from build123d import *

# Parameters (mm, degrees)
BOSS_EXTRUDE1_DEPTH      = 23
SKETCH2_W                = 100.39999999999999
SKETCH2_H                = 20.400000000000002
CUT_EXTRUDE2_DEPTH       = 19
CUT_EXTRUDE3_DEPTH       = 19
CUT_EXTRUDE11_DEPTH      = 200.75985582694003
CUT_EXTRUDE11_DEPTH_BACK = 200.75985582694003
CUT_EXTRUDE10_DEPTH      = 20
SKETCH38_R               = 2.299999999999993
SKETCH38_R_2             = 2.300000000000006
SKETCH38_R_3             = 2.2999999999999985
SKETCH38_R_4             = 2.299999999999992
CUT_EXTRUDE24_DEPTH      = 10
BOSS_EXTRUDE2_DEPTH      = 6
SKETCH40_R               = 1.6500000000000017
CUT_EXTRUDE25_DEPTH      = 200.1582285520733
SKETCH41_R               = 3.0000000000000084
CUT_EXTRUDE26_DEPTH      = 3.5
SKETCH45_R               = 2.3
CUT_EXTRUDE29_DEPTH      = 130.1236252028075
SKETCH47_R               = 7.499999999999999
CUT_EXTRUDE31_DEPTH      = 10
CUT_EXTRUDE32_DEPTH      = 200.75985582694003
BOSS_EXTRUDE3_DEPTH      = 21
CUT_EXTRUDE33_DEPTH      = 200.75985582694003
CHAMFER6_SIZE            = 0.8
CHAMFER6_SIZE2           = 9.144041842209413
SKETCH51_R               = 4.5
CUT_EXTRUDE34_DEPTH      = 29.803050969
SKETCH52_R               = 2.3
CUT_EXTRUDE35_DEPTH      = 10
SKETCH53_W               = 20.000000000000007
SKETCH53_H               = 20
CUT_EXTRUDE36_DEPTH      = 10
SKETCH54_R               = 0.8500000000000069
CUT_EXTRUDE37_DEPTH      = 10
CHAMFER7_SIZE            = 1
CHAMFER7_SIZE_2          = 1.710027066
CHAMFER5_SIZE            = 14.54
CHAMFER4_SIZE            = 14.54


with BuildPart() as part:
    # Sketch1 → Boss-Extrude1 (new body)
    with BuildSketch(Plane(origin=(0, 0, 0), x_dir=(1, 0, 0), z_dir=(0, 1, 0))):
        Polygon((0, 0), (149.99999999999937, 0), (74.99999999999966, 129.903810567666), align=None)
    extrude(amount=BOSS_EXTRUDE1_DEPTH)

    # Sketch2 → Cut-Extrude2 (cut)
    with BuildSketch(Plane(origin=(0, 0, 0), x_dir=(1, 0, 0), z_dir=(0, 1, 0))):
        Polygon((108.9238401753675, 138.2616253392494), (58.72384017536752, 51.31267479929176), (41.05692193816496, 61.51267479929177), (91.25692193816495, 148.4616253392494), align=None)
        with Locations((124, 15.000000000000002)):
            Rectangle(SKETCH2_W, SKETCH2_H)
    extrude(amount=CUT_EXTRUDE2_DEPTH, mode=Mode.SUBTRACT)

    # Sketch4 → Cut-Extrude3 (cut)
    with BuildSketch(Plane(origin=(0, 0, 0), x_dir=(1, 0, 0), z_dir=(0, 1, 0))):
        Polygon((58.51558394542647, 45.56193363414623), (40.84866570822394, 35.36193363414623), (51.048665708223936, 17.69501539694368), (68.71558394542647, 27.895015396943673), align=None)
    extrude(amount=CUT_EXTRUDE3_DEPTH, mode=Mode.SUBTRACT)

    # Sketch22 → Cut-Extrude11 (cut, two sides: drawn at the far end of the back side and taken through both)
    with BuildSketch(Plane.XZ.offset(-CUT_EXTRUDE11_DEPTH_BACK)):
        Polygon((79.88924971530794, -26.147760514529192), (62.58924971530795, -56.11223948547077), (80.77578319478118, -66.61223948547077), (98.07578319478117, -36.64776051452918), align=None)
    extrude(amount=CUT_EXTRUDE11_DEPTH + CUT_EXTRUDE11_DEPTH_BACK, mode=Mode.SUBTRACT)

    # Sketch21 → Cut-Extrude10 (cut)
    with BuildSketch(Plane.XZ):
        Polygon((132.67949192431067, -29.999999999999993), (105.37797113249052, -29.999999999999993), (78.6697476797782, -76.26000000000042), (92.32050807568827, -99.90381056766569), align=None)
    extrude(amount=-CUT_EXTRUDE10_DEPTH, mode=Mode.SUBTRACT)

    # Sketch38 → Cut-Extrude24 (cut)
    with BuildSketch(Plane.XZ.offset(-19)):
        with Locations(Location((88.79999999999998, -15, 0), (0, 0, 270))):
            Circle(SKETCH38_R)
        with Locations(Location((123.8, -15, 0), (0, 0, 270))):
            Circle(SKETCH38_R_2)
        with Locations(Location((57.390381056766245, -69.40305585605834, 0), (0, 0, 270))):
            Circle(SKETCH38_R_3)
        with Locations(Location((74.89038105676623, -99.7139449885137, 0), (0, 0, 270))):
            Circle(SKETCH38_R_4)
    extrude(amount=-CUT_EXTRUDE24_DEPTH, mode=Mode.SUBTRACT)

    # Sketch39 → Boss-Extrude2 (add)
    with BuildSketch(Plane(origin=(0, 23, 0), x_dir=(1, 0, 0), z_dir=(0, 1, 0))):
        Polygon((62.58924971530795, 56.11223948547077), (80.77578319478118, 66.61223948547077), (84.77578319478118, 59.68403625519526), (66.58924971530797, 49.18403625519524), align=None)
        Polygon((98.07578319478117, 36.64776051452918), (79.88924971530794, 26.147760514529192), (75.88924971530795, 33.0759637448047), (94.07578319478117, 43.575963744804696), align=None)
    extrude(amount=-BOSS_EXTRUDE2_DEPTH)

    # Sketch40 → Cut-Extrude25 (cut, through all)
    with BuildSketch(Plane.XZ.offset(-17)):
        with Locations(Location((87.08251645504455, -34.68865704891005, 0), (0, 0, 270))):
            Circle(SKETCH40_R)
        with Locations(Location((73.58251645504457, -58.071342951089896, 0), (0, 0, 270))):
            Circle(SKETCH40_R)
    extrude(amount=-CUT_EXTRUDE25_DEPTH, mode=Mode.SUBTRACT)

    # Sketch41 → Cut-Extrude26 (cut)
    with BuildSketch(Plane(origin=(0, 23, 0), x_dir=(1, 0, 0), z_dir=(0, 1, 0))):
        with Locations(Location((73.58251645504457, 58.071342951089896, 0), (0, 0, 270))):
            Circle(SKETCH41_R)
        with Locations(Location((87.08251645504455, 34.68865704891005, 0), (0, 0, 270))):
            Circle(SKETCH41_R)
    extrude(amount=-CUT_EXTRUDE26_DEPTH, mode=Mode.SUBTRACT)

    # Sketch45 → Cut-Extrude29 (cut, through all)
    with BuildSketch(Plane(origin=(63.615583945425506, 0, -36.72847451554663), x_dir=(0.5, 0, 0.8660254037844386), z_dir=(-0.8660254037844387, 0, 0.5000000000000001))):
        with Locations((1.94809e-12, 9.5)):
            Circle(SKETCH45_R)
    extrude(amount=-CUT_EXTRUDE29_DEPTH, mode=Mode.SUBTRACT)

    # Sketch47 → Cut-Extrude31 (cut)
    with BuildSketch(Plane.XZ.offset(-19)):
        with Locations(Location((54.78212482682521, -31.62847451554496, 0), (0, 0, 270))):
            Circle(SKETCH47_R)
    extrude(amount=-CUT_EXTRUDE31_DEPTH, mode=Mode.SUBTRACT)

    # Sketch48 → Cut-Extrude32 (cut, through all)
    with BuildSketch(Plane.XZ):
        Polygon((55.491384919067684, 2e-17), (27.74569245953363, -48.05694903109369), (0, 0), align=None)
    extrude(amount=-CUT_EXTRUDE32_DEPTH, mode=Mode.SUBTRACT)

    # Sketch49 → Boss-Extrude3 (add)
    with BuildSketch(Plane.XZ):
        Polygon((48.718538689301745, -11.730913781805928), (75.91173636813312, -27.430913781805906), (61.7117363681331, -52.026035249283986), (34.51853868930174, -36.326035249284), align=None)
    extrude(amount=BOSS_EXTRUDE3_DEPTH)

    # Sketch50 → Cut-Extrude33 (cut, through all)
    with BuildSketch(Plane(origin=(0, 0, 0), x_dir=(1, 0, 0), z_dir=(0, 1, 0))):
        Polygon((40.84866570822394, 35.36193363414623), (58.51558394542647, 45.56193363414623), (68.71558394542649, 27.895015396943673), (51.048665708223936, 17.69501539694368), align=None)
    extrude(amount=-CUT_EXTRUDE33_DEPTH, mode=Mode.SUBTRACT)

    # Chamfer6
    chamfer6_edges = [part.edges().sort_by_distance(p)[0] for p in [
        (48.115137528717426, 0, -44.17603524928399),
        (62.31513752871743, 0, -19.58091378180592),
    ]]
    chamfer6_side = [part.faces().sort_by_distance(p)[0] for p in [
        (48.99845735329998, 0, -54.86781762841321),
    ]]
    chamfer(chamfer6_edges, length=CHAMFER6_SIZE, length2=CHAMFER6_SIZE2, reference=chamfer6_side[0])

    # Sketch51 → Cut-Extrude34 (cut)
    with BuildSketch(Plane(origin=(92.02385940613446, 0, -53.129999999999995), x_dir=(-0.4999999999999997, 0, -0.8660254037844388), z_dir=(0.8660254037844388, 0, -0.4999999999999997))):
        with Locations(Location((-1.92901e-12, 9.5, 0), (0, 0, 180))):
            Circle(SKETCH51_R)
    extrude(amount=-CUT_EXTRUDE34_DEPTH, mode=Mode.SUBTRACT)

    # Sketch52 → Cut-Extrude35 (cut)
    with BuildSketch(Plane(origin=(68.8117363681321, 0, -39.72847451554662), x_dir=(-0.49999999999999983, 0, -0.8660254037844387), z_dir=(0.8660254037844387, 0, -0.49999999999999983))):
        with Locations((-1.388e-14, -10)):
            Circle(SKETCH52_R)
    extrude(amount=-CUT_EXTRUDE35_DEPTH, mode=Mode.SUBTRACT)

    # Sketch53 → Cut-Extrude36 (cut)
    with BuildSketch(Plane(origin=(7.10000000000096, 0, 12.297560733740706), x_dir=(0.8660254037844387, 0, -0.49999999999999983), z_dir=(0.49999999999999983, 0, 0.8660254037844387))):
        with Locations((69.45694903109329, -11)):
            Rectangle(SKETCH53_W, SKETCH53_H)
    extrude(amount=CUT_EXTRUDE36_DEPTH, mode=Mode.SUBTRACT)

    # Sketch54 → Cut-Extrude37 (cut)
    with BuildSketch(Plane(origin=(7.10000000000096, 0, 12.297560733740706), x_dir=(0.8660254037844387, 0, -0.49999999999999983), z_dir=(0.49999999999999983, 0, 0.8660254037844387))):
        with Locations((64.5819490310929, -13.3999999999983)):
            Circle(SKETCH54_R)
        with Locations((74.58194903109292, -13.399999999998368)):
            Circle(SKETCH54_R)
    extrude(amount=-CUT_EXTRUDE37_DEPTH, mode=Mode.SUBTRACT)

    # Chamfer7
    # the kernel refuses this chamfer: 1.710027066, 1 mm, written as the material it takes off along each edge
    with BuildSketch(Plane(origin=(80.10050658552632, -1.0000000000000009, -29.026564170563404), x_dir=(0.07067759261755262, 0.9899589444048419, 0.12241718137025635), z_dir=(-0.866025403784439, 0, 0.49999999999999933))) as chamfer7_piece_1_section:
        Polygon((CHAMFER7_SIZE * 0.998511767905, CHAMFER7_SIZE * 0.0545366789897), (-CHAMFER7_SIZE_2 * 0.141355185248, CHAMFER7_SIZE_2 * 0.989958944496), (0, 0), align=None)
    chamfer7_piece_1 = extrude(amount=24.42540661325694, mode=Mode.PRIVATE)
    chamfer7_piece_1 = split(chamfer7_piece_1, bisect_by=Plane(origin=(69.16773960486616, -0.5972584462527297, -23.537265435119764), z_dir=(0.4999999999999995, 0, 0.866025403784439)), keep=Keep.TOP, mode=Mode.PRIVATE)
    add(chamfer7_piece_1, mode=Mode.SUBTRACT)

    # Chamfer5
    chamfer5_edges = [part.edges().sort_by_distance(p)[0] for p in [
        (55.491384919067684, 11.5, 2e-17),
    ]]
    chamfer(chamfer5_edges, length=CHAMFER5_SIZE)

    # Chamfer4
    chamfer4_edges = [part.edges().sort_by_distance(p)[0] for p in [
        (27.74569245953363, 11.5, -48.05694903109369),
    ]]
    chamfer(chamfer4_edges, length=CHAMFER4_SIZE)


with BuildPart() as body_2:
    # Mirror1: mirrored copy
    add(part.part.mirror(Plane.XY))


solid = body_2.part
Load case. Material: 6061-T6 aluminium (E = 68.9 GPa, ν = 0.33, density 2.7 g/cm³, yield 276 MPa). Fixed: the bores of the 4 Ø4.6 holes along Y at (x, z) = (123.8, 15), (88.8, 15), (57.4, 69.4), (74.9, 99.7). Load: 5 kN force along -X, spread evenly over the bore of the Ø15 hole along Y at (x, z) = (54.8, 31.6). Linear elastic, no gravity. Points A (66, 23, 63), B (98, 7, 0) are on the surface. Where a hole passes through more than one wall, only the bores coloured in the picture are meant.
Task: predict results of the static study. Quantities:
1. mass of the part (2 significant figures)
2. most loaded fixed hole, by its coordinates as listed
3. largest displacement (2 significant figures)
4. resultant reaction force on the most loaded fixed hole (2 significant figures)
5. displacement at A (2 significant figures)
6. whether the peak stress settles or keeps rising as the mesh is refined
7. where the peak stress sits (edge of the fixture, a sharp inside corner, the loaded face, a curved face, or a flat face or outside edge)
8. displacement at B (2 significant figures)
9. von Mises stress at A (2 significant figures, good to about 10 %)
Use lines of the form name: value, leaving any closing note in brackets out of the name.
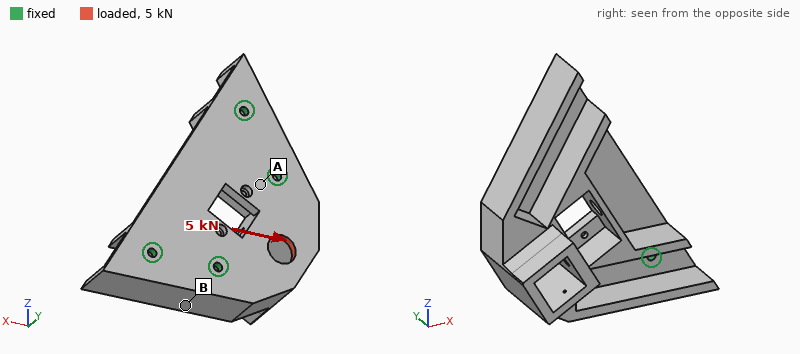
mass of the part: 240 g
most loaded fixed hole, by its coordinates as listed: (88.8, 15)
largest displacement: 25 µm
resultant reaction force on the most loaded fixed hole: 2.6 kN
displacement at A: 4.9 µm
whether the peak stress settles or keeps rising as the mesh is refined: keeps rising
where the peak stress sits: edge of the fixture
displacement at B: 4.9 µm
von Mises stress at A: 12 MPa
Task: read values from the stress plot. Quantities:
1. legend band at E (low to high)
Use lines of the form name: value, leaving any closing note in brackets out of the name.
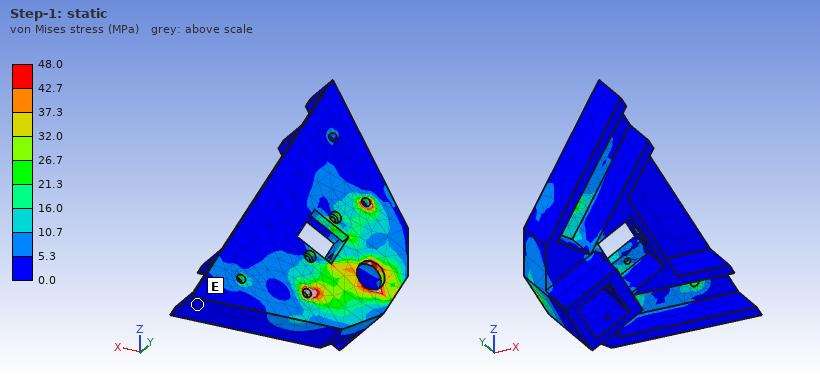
legend band at E: 0.0 to 5.3 MPa
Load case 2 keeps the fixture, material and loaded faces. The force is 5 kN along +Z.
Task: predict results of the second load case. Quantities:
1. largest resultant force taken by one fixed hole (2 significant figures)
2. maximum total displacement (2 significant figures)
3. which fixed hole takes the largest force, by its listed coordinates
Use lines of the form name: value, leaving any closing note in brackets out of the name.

largest resultant force taken by one fixed hole: 2.8 kN
maximum total displacement: 25 µm
which fixed hole takes the largest force, by its listed coordinates: (57.4, 69.4)
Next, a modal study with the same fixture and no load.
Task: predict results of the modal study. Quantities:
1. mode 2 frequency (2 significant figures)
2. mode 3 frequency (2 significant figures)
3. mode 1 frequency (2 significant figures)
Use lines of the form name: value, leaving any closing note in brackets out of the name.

mode 2 frequency: 3900 Hz
mode 3 frequency: 4000 Hz
mode 1 frequency: 2500 Hz
